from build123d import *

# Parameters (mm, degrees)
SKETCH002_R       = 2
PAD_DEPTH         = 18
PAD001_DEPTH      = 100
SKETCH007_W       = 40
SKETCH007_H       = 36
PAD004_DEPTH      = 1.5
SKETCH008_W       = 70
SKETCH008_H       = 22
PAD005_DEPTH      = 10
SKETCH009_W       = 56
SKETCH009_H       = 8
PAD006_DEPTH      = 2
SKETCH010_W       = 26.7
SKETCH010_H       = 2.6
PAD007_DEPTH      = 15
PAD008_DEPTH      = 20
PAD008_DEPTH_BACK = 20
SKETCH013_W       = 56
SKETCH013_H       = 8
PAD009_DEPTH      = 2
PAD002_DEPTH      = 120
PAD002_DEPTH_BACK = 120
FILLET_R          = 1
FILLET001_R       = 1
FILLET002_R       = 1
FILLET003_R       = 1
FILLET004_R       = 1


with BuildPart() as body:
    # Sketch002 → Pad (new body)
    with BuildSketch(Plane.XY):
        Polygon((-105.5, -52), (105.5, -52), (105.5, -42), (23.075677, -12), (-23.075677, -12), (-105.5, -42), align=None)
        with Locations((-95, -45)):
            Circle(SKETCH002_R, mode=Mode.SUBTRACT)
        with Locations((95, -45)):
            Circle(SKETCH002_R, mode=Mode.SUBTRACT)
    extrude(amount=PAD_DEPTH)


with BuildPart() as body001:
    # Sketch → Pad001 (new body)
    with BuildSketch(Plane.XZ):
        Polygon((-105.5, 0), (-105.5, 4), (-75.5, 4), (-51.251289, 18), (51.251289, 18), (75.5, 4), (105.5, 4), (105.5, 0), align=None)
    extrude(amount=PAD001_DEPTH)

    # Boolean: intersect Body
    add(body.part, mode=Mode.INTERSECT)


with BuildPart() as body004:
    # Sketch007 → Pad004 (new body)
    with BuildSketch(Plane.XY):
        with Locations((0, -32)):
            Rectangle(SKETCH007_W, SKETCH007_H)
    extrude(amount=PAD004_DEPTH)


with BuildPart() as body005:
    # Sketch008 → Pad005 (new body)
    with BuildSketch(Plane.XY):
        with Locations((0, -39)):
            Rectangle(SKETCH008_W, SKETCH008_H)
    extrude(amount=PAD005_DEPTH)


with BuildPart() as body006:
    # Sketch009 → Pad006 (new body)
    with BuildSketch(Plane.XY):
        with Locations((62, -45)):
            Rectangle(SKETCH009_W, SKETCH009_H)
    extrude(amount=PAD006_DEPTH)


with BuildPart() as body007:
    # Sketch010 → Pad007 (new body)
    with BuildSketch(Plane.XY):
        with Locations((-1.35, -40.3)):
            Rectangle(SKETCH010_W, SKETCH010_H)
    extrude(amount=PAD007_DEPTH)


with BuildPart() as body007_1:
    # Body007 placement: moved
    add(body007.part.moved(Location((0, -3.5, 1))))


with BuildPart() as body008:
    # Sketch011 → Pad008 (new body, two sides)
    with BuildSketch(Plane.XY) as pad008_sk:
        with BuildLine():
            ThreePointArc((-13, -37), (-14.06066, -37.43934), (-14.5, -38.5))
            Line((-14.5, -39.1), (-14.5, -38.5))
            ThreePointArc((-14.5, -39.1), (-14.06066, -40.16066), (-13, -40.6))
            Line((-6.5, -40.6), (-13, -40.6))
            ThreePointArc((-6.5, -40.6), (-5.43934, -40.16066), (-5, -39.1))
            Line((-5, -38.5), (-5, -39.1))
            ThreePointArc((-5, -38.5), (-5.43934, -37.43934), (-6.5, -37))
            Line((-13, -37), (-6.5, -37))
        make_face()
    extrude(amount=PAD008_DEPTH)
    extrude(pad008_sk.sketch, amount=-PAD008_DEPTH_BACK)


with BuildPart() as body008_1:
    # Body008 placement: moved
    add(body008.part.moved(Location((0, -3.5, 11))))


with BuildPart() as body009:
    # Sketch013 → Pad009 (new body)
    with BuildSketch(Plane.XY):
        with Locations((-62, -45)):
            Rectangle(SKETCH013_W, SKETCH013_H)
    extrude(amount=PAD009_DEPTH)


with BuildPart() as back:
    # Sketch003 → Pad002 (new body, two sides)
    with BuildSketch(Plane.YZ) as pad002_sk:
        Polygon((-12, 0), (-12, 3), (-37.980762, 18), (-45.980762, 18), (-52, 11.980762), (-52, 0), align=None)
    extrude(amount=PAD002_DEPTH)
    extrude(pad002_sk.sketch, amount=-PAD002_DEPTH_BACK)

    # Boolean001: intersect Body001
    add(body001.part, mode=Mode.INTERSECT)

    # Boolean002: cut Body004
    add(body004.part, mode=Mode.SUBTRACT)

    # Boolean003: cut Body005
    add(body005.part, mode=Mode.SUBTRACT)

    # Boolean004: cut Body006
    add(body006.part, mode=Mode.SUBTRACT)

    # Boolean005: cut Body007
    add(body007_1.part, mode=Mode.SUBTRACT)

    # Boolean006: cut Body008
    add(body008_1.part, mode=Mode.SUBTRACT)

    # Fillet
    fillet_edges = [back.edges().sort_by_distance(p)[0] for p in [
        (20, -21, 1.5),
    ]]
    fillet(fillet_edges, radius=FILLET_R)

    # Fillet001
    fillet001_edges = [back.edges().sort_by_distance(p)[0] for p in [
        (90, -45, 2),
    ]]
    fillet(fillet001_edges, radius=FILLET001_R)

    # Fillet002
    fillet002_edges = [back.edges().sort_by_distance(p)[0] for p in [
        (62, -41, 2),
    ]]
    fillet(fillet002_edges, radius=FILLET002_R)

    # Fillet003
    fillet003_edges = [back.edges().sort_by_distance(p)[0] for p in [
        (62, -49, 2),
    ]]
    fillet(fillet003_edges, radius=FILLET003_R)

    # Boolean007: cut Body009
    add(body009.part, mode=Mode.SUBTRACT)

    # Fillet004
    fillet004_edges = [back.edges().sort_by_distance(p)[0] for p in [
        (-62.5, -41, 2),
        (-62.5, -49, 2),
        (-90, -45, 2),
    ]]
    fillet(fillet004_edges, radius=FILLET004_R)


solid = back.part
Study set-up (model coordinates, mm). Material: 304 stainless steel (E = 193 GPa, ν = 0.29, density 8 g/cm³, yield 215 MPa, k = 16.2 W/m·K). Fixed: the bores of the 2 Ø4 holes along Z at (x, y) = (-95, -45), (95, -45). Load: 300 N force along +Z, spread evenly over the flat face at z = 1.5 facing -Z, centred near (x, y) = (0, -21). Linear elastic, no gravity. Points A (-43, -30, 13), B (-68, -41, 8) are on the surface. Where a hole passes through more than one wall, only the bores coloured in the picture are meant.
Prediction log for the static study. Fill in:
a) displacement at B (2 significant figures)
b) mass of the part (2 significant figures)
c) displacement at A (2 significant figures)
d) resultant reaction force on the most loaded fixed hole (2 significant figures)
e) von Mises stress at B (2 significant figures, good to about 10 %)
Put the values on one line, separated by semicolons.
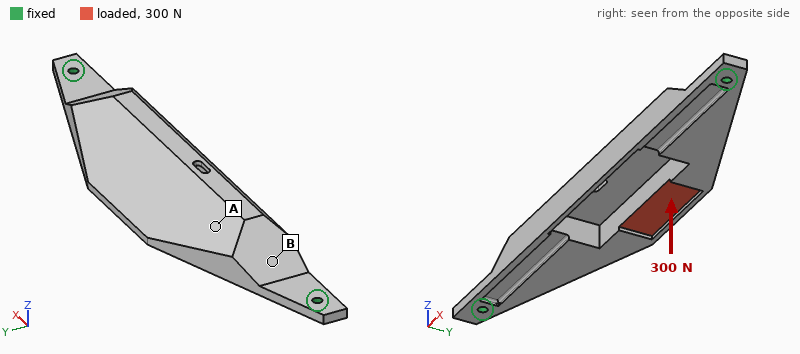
0.036 mm; 390 g; 0.092 mm; 580 N; 20 MPa
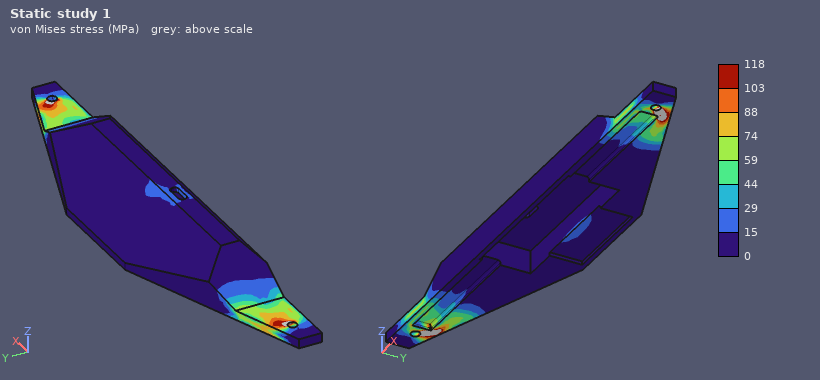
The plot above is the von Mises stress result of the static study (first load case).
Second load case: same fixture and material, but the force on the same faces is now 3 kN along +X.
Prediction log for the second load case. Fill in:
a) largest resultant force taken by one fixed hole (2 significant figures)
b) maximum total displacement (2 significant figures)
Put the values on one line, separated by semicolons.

1.5 kN; 31 µm
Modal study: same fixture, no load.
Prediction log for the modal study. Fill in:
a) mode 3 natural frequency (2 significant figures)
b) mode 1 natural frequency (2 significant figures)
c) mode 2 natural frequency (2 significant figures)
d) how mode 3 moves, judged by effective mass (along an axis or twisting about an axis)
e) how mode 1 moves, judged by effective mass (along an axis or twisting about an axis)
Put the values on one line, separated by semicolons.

2100 Hz; 670 Hz; 1300 Hz; twisting about Y; along Z
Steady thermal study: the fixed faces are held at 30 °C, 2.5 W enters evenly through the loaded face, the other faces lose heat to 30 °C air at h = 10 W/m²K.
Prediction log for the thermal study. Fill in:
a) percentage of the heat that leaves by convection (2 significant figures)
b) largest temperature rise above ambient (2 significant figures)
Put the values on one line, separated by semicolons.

77 %; 22 K
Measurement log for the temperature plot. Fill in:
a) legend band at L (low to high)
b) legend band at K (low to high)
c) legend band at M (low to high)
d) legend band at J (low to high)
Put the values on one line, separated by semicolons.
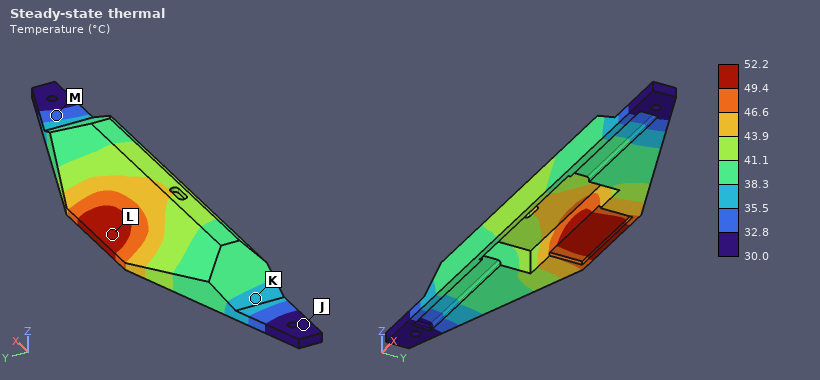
49.4 to 52.2 °C; 35.5 to 38.3 °C; 32.8 to 35.5 °C; 30.0 to 32.8 °C
